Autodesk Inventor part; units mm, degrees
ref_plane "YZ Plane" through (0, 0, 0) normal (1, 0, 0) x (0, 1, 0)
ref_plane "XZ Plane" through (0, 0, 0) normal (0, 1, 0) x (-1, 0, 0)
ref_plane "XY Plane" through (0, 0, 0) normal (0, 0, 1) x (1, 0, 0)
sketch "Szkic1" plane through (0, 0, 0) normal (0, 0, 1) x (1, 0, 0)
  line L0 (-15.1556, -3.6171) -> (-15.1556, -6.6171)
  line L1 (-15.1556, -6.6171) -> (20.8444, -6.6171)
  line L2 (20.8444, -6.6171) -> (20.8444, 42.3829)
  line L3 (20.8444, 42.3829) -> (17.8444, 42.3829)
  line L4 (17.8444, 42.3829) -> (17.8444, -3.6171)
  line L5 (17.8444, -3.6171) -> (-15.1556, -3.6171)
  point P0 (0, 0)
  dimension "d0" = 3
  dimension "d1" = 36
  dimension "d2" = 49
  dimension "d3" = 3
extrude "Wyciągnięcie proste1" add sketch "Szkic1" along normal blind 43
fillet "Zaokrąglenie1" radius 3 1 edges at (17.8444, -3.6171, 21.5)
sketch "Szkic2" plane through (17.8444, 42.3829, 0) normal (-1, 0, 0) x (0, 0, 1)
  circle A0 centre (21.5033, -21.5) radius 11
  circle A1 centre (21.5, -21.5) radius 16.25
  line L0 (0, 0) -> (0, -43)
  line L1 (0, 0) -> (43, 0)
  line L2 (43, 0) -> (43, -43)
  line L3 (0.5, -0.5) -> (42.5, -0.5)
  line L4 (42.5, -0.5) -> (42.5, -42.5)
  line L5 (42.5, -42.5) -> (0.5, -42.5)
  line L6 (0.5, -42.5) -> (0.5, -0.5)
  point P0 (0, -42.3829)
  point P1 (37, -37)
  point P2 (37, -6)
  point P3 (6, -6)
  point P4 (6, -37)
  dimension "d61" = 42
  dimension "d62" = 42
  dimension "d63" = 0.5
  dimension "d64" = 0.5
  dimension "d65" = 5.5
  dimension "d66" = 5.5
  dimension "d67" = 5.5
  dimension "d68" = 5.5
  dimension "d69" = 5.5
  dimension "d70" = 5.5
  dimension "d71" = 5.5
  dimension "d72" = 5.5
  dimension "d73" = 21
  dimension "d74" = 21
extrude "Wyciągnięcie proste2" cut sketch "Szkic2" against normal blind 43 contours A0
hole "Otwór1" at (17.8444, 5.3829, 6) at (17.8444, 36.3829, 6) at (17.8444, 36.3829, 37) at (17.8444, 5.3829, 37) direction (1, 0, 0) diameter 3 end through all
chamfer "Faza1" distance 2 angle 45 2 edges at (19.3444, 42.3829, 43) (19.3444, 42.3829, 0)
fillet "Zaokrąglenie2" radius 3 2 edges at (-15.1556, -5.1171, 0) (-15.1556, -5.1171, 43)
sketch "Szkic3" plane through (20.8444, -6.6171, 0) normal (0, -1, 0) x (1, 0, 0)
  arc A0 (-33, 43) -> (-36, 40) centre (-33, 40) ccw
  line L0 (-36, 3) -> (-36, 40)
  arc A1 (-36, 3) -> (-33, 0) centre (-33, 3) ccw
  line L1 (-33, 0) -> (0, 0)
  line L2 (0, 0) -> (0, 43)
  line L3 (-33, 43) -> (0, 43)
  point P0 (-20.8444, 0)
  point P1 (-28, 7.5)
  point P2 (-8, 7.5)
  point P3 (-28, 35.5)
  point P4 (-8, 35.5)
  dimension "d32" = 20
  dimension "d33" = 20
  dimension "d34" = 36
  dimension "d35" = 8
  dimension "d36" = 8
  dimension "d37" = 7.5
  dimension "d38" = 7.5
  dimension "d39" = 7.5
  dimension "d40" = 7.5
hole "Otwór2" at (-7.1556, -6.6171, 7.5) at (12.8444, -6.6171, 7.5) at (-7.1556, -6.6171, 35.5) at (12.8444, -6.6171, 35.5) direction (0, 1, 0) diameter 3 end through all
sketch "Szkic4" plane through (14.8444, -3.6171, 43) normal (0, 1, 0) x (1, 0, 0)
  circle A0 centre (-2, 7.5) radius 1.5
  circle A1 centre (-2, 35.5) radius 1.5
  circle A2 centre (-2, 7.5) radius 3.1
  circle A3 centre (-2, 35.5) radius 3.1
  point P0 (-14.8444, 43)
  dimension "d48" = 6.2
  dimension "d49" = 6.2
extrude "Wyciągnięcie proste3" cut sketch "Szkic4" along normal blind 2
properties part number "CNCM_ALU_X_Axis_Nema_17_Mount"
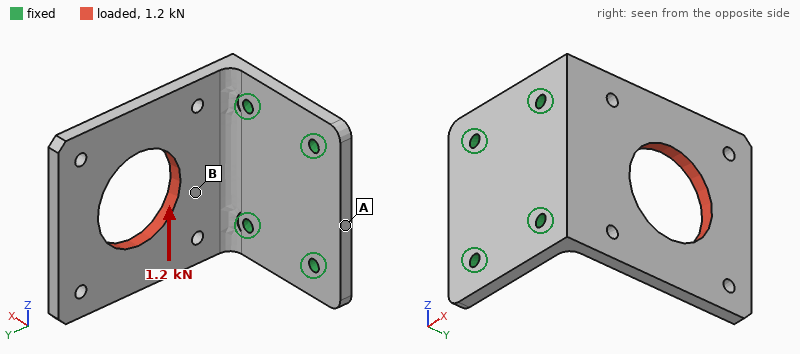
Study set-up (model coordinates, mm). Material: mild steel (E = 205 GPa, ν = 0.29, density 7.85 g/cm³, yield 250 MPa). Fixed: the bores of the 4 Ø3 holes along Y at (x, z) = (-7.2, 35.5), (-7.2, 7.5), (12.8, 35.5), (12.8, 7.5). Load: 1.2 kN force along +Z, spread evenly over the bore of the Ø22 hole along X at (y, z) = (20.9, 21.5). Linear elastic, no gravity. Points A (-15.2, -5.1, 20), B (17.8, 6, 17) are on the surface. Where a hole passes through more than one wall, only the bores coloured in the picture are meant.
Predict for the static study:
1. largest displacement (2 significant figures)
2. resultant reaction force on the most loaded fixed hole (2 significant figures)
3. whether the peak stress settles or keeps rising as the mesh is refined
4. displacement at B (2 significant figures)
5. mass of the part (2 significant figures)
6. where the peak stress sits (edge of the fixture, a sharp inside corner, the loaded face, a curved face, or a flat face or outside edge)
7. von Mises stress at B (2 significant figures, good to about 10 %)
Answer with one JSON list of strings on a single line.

["59 µm", "1.2 kN", "keeps rising", "12 µm", "73 g", "edge of the fixture", "55 MPa"]
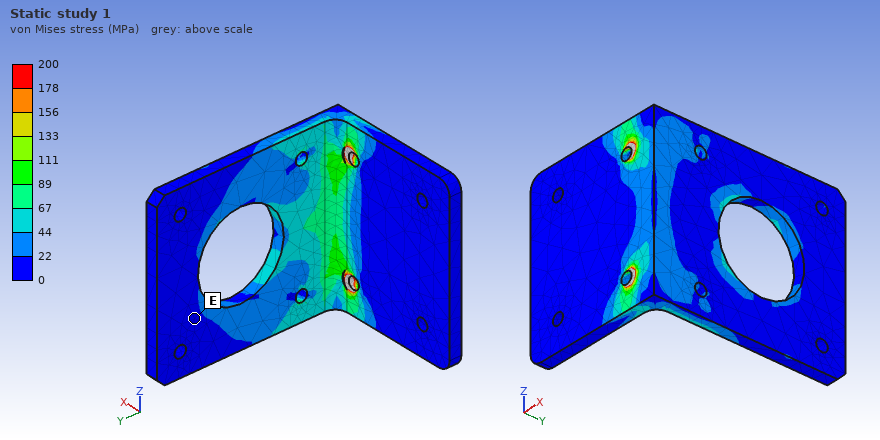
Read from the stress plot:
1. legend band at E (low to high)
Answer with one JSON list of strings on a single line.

["0 to 22 MPa"]
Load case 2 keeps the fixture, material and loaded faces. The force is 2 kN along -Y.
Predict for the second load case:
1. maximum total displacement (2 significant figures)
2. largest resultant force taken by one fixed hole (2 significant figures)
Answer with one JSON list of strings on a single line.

["0.11 mm", "1.1 kN"]
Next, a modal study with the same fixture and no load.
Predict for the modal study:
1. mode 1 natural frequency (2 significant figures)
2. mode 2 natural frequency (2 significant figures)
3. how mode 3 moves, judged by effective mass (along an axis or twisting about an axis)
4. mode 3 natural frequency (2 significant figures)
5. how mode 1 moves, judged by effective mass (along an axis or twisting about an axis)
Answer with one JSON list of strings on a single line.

["970 Hz", "2500 Hz", "along Z", "4900 Hz", "along X"]
